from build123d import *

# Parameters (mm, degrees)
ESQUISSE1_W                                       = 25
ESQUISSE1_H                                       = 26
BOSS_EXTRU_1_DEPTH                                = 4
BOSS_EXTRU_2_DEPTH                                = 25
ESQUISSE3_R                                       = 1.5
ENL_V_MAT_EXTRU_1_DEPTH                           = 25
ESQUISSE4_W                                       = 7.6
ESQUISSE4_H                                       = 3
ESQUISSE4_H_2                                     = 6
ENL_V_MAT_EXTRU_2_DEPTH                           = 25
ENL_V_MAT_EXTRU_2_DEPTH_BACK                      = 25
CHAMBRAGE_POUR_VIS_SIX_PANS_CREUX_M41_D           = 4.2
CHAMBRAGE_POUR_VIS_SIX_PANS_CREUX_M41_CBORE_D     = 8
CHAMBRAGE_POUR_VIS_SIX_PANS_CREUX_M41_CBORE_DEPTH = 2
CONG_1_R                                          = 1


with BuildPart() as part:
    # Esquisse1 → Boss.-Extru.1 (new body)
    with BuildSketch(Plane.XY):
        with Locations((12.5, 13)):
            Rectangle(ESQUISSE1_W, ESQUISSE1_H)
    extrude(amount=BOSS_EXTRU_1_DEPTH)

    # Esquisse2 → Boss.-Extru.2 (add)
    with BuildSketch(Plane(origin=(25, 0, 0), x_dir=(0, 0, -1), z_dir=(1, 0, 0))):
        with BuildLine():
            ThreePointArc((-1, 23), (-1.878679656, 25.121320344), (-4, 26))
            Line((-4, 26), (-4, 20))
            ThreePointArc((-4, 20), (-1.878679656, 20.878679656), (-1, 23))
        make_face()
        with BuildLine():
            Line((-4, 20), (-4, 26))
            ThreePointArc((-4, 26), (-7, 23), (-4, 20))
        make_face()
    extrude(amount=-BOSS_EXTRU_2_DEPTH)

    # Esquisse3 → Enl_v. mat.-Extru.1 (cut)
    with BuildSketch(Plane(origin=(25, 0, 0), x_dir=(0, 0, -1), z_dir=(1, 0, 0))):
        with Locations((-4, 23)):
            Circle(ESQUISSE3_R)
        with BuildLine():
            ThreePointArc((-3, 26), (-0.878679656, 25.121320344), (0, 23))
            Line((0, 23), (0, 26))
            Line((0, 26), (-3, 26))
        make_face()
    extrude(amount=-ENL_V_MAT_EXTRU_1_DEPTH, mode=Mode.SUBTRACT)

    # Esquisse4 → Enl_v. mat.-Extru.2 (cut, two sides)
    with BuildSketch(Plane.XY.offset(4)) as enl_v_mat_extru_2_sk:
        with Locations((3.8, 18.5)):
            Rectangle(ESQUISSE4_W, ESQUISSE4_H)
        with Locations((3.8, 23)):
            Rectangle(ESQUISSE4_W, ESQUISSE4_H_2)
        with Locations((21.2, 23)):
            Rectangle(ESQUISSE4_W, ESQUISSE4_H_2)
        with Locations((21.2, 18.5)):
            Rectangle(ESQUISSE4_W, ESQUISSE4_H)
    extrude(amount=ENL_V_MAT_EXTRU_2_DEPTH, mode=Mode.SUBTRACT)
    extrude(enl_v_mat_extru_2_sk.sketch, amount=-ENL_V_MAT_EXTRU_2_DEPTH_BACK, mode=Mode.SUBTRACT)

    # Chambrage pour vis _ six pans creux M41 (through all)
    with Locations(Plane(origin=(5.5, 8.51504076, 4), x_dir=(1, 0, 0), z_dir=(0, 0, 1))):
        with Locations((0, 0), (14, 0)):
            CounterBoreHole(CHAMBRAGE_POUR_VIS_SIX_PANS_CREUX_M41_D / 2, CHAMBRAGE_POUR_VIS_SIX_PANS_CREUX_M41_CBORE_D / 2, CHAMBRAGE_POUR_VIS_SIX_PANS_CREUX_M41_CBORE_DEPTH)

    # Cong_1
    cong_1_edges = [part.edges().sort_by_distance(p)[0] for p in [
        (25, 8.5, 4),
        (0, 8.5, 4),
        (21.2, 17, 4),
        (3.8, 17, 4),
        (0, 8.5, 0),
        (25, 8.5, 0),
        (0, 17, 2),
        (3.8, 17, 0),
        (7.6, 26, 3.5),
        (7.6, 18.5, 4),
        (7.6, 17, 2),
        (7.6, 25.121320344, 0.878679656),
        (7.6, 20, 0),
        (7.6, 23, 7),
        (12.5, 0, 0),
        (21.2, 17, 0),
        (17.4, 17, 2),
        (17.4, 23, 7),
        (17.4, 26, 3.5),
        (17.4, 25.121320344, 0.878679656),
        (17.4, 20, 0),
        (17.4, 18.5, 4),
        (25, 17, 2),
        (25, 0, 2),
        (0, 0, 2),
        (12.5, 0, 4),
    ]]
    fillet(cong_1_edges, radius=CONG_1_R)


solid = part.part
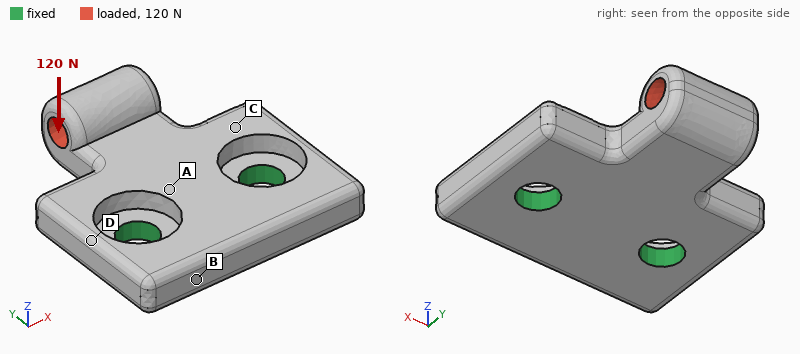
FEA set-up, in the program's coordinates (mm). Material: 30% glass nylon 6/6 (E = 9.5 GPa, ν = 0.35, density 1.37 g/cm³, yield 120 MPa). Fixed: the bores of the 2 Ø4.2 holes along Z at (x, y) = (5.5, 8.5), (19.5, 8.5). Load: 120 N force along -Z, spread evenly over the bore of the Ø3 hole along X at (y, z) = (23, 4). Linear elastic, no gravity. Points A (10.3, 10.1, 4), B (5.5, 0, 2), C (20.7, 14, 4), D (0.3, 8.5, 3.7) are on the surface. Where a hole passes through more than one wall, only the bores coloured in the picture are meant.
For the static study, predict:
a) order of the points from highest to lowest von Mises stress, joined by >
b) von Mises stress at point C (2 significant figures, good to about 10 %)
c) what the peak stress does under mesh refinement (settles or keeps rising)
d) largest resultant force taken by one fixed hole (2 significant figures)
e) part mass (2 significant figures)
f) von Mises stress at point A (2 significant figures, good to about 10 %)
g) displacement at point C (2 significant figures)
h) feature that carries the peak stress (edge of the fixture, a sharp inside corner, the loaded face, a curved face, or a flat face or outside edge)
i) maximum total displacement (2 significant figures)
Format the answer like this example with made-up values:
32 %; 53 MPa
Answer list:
A > C > D > B; 23 MPa; keeps rising; 79 N; 2.5 g; 32 MPa; 0.051 mm; edge of the fixture; 0.32 mm
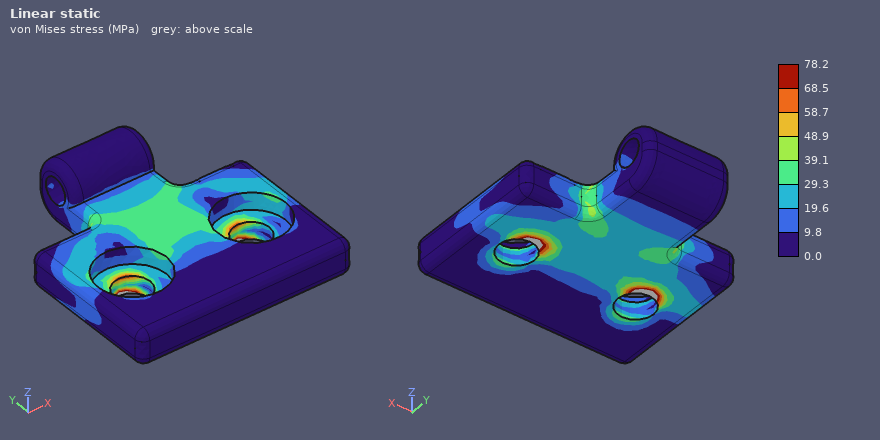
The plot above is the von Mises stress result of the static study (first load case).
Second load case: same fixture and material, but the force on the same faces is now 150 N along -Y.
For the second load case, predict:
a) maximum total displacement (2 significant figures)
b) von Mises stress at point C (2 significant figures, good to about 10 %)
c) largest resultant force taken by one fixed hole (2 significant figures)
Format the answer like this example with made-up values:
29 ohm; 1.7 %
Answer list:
0.11 mm; 7.7 MPa; 76 N
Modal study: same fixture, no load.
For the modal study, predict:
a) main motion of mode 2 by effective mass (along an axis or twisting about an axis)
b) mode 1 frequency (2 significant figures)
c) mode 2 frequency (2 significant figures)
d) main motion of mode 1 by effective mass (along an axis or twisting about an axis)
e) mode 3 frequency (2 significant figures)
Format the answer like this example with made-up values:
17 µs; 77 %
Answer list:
along Z; 5000 Hz; 15 kHz; along Z; 16 kHz
